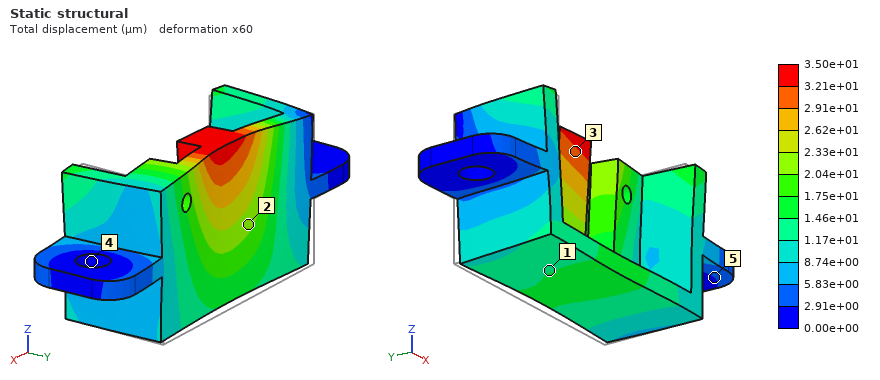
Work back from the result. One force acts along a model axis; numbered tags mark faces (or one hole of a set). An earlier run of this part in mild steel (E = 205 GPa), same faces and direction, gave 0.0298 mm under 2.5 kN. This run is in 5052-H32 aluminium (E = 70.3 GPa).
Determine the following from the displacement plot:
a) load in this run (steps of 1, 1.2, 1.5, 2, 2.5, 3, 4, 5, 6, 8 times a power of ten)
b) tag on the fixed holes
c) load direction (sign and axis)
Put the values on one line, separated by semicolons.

1 kN; 4; -Y
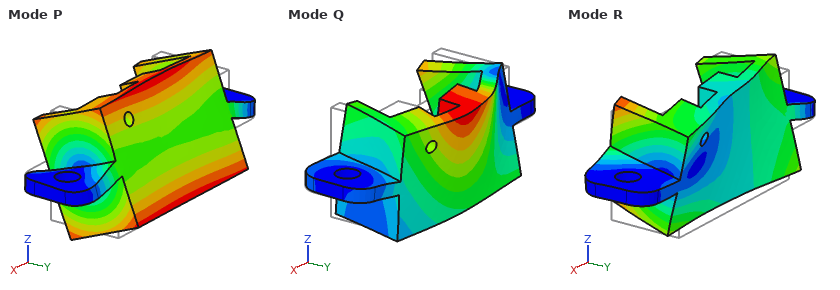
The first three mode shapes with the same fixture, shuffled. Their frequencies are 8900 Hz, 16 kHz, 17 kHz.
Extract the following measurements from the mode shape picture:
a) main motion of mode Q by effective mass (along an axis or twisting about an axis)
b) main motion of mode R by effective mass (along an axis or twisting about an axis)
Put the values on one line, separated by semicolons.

along Y; along Z
